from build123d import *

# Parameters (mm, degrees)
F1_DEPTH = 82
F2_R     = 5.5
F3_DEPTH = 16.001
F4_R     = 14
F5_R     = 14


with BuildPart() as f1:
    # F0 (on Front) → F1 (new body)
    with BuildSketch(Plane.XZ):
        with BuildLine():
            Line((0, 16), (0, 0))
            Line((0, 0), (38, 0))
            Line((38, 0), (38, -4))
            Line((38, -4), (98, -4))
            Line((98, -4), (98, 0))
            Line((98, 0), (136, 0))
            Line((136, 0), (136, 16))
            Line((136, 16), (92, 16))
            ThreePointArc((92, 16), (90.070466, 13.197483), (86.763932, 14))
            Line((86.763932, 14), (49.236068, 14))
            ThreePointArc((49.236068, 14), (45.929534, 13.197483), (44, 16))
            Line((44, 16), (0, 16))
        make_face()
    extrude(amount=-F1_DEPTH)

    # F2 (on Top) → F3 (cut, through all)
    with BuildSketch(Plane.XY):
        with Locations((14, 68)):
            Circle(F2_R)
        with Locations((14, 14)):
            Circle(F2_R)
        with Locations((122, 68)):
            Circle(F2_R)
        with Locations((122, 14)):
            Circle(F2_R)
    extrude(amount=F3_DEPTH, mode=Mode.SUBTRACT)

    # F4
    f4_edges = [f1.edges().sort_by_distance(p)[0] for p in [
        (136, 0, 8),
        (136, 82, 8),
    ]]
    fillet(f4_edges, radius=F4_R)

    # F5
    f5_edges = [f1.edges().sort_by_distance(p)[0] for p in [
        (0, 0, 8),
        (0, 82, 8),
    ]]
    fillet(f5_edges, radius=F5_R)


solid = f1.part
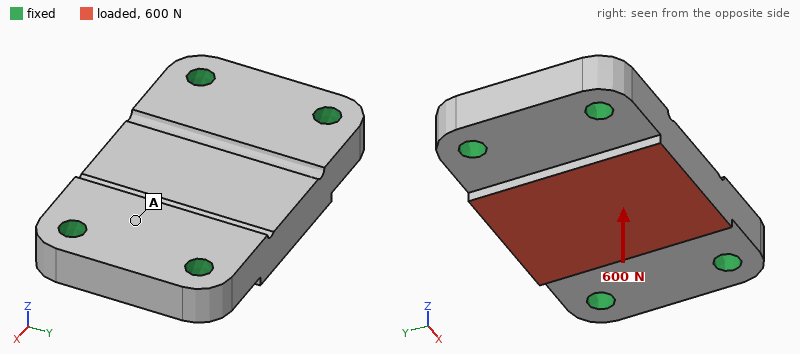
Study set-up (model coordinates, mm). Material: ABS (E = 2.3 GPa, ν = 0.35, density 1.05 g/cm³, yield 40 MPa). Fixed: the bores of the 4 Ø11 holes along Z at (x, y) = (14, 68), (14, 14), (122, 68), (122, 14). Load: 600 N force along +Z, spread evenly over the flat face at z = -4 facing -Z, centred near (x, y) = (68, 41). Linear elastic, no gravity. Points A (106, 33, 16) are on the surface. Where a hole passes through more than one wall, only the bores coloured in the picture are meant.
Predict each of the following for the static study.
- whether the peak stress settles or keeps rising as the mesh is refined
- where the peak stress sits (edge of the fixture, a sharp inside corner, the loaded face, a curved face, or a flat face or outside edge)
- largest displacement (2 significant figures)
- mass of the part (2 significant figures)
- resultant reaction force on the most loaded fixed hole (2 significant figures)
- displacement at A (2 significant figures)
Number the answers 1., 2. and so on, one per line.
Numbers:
1. keeps rising
2. edge of the fixture
3. 51 µm
4. 190 g
5. 180 N
6. 19 µm
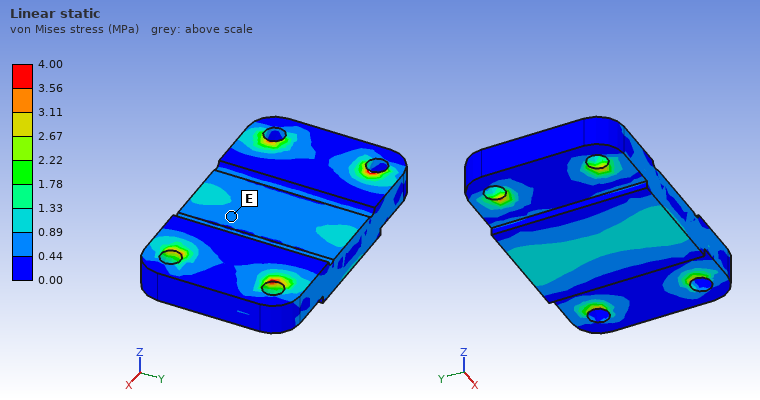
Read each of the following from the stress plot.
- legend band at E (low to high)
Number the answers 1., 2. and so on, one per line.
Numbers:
1. 0.44 to 0.89 MPa
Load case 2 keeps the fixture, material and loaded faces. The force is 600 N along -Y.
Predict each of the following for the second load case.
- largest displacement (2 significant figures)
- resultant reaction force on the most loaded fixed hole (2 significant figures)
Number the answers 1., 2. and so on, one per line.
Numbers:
1. 33 µm
2. 200 N
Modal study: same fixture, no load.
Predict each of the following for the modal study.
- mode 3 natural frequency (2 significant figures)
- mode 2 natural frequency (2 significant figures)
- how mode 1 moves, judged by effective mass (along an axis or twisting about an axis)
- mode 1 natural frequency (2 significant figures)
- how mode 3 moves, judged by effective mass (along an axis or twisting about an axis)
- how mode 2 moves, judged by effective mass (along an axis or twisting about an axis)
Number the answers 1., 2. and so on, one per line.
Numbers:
1. 3500 Hz
2. 2400 Hz
3. along Z
4. 1900 Hz
5. along Y
6. twisting about X
